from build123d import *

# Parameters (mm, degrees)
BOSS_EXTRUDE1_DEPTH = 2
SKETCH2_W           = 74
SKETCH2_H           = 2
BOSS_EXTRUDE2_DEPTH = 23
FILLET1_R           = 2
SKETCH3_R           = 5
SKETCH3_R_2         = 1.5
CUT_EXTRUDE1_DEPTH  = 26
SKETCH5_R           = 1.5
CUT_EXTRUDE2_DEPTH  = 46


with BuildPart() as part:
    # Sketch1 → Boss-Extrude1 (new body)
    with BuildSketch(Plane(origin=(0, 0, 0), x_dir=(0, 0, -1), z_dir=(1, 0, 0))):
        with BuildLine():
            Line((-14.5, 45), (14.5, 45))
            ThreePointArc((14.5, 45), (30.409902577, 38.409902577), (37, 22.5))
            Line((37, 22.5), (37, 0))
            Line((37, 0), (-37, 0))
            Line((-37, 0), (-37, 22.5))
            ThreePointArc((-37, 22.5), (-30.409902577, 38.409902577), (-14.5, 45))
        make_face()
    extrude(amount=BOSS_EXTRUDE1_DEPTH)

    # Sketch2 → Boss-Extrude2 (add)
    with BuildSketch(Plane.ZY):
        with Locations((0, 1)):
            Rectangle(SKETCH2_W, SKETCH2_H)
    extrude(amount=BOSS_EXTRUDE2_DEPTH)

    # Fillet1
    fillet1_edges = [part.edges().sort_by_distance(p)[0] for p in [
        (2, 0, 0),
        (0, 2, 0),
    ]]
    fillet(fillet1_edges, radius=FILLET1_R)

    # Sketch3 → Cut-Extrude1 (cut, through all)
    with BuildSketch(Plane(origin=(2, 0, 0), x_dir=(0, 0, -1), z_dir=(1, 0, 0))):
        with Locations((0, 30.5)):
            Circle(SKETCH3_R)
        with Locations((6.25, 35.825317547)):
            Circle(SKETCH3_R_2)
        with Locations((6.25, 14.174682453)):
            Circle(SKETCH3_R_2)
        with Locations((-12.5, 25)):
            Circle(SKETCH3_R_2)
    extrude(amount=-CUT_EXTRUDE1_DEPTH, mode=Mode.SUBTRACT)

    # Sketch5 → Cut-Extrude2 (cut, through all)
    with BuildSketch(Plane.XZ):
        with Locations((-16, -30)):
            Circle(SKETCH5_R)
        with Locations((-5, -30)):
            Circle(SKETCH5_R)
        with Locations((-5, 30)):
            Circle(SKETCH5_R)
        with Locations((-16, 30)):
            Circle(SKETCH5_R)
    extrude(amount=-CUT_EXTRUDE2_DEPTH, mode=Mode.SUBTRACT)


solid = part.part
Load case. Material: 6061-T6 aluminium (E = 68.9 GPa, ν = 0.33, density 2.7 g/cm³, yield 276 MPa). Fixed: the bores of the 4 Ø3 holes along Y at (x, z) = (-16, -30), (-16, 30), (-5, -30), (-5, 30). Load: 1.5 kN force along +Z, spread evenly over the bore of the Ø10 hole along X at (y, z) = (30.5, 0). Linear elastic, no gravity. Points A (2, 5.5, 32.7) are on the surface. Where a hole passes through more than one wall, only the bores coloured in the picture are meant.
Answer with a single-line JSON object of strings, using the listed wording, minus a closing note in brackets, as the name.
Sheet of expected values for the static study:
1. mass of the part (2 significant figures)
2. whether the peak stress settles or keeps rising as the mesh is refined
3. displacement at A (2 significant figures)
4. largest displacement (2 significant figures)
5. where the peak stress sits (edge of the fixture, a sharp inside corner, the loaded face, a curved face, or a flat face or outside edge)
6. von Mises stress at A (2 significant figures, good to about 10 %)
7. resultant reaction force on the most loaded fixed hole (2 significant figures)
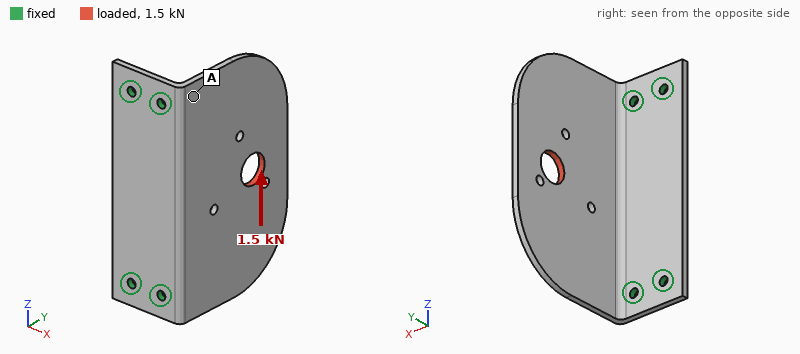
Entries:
{"mass of the part": "25 g", "whether the peak stress settles or keeps rising as the mesh is refined": "keeps rising", "displacement at A": "0.085 mm", "largest displacement": "0.23 mm", "where the peak stress sits": "edge of the fixture", "von Mises stress at A": "37 MPa", "resultant reaction force on the most loaded fixed hole": "1000 N"}
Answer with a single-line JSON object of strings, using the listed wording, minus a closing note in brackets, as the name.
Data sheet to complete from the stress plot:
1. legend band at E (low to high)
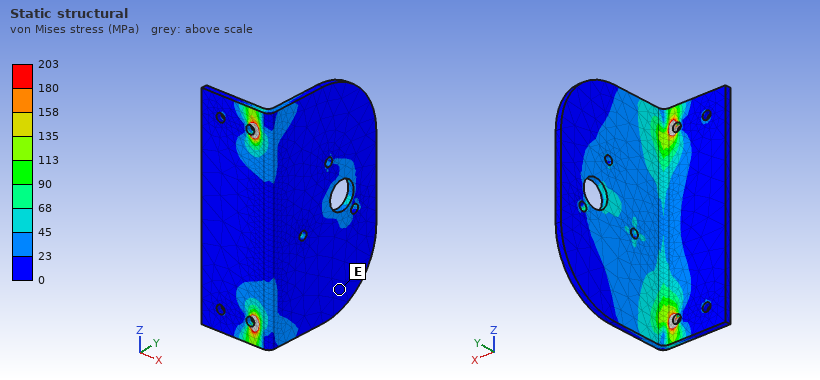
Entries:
{"legend band at E": "0 to 23 MPa"}
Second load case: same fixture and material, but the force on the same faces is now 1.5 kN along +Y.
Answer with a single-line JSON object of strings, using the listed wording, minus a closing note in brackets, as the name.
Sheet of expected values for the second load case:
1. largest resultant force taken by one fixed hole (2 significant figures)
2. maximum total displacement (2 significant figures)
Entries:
{"largest resultant force taken by one fixed hole": "940 N", "maximum total displacement": "0.46 mm"}
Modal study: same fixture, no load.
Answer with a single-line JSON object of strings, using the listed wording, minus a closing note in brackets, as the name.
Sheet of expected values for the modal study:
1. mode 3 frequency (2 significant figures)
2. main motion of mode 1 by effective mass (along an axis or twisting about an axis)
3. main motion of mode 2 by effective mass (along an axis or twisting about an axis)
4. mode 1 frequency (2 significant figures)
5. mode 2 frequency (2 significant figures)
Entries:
{"mode 3 frequency": "3400 Hz", "main motion of mode 1 by effective mass": "along X", "main motion of mode 2 by effective mass": "twisting about Y", "mode 1 frequency": "780 Hz", "mode 2 frequency": "1600 Hz"}
